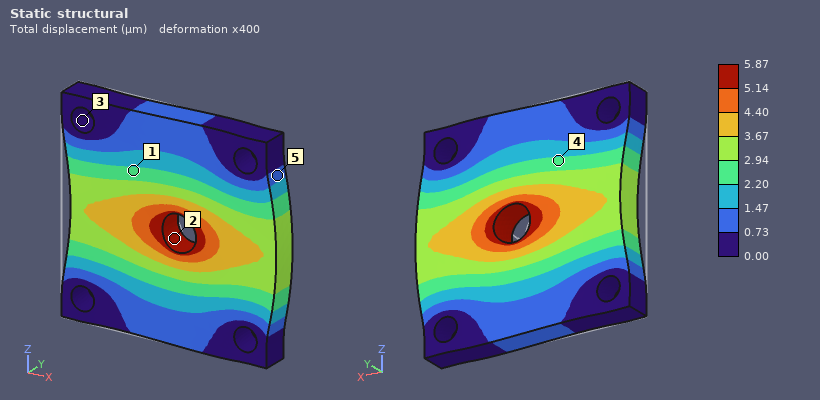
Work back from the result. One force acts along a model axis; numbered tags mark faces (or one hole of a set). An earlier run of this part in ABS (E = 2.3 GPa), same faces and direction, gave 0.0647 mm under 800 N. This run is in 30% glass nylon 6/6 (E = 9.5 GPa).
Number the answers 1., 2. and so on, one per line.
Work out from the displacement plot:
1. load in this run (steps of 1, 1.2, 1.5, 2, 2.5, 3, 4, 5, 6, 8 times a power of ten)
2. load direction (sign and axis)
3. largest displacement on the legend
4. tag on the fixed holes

1. 300 N
2. +X
3. 5.87 µm
4. 3
